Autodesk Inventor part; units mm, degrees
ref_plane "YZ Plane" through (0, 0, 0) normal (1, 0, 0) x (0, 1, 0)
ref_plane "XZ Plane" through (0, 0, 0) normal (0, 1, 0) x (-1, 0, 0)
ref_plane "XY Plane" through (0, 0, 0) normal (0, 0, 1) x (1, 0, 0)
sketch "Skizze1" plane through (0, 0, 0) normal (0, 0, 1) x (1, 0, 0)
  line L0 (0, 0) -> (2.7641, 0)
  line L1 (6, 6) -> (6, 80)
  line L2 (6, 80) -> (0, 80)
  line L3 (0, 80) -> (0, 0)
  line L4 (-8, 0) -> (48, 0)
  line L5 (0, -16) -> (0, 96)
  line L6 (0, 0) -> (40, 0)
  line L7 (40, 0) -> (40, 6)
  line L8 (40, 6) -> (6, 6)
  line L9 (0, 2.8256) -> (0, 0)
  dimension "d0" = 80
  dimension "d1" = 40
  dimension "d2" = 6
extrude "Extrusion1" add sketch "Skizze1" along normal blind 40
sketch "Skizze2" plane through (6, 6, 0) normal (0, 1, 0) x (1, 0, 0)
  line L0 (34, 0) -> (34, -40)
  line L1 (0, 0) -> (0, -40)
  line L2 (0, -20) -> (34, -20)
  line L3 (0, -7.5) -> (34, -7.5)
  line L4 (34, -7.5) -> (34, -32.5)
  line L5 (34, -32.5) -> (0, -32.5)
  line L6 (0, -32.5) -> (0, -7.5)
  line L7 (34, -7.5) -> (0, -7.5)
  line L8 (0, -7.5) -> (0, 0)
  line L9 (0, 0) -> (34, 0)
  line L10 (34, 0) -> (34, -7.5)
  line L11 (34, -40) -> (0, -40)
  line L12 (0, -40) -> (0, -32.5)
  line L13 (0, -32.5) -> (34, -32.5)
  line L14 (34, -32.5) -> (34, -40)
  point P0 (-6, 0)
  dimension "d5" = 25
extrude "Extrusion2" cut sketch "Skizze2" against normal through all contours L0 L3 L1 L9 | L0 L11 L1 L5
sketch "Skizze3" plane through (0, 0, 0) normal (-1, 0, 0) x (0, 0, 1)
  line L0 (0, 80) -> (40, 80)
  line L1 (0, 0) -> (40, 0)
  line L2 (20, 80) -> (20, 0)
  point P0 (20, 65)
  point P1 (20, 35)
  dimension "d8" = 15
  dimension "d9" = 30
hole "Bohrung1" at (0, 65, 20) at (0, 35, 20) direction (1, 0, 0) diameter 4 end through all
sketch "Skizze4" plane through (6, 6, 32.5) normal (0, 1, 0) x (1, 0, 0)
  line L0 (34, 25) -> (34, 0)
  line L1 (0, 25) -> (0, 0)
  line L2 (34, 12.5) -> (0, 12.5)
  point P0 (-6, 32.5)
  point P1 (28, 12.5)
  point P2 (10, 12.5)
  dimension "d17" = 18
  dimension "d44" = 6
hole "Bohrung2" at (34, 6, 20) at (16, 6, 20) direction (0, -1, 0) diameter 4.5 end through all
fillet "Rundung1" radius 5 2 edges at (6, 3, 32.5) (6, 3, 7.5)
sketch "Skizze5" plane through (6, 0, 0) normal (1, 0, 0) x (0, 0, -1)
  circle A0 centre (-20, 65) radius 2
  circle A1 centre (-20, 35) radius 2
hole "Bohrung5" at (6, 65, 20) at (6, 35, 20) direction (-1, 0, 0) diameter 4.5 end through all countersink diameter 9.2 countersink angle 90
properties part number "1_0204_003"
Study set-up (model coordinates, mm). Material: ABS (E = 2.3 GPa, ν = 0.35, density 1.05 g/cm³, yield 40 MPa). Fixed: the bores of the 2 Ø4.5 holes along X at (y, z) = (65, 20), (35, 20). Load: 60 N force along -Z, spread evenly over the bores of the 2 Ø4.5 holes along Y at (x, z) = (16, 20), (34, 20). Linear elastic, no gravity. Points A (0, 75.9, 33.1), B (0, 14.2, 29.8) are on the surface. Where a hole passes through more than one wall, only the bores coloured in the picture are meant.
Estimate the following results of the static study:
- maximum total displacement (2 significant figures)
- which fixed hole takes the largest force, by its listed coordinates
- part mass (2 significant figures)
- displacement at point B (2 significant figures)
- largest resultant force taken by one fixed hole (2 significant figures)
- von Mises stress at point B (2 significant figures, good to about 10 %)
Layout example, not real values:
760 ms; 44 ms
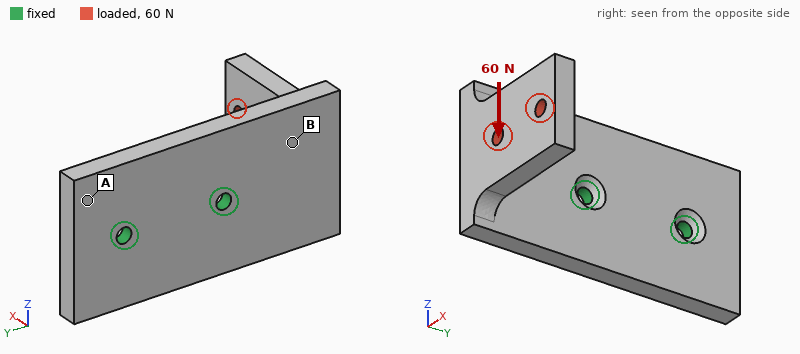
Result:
0.98 mm; (35, 20); 25 g; 0.18 mm; 110 N; 3.5 MPa
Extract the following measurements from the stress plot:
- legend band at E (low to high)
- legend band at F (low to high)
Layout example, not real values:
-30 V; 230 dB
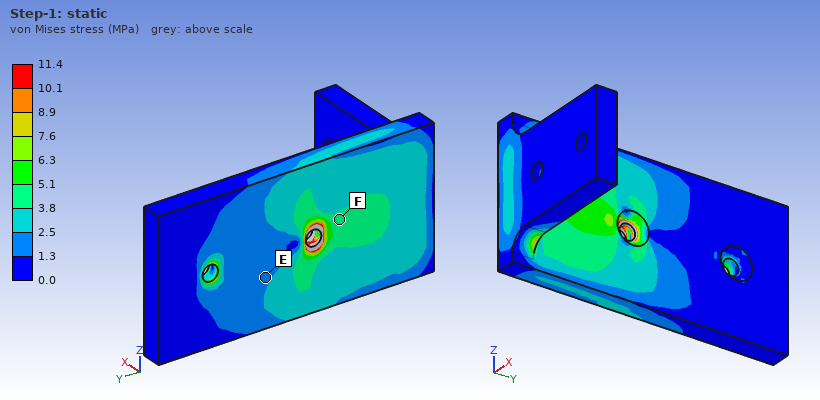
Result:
1.3 to 2.5 MPa; 3.8 to 5.1 MPa
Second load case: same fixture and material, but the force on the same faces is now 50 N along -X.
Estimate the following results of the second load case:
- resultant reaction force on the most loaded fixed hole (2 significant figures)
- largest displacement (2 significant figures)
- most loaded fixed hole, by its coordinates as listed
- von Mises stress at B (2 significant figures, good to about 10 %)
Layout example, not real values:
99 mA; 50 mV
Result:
95 N; 0.91 mm; (35, 20); 2.2 MPa
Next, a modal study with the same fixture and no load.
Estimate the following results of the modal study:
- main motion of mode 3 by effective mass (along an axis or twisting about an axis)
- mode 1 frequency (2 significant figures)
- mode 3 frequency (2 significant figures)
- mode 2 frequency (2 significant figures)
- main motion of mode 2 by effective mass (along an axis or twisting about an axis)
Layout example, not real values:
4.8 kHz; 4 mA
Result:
along X; 440 Hz; 1100 Hz; 620 Hz; along Z
